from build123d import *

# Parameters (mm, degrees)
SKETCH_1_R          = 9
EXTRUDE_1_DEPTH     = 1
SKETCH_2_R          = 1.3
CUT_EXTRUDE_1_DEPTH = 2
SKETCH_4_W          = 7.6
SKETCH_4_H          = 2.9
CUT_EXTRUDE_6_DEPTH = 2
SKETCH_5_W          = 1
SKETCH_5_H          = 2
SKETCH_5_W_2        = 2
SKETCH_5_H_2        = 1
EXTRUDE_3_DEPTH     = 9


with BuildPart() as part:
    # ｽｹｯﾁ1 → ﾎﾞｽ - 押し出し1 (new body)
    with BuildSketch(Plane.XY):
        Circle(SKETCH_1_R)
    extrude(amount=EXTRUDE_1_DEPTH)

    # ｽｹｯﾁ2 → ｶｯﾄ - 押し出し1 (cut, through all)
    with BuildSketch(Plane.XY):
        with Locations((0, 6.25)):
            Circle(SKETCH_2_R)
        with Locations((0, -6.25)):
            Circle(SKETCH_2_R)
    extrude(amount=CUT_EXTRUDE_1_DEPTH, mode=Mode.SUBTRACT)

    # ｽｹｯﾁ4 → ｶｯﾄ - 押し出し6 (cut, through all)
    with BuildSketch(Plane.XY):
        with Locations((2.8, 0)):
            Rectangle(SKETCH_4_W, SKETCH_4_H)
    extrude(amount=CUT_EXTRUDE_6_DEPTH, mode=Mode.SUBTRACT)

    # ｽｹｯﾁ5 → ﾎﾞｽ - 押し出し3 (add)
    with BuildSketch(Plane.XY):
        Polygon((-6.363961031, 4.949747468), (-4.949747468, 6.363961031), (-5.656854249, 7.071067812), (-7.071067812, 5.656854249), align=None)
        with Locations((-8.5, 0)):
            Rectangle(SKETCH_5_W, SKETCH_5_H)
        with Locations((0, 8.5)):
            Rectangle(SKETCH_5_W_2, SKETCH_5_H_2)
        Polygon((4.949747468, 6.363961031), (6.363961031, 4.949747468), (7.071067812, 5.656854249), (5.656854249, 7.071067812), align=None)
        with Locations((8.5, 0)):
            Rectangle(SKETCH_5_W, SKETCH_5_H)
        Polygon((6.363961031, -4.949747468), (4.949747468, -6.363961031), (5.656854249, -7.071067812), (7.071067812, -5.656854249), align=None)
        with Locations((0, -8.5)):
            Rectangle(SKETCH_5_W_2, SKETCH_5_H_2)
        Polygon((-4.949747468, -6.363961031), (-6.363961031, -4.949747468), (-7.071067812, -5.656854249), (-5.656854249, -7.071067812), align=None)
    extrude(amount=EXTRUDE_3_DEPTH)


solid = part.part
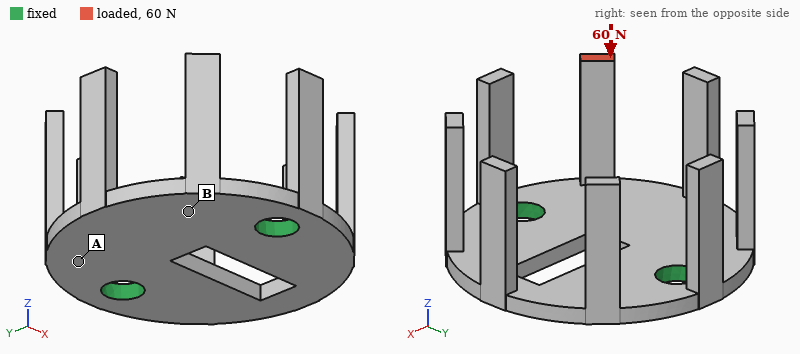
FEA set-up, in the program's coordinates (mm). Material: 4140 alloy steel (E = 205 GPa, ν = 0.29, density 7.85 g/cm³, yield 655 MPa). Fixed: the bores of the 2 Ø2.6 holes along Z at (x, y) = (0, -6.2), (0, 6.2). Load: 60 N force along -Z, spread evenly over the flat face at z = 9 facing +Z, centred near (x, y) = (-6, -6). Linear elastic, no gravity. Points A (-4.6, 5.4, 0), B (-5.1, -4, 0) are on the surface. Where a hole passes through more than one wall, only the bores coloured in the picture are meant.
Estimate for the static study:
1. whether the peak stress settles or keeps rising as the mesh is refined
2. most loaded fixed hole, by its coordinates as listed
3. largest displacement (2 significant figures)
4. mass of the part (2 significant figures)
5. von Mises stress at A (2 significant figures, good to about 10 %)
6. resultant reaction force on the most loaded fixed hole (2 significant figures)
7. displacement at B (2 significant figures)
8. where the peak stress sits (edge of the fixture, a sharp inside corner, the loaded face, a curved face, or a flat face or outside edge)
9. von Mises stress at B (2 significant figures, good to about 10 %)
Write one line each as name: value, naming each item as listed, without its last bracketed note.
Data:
whether the peak stress settles or keeps rising as the mesh is refined: keeps rising
most loaded fixed hole, by its coordinates as listed: (0, -6.2)
largest displacement: 53 µm
mass of the part: 2.7 g
von Mises stress at A: 34 MPa
resultant reaction force on the most loaded fixed hole: 59 N
displacement at B: 13 µm
where the peak stress sits: edge of the fixture
von Mises stress at B: 76 MPa
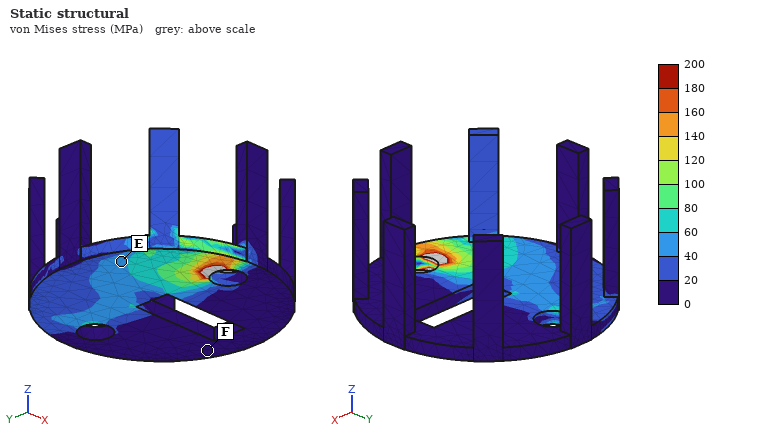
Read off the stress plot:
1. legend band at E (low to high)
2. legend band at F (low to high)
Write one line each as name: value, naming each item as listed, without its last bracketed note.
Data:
legend band at E: 40 to 60 MPa
legend band at F: 0 to 20 MPa
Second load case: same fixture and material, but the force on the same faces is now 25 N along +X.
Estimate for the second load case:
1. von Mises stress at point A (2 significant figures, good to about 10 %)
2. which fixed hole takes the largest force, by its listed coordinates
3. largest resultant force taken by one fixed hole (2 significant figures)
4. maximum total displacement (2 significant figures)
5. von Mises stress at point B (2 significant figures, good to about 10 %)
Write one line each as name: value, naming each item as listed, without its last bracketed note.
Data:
von Mises stress at point A: 39 MPa
which fixed hole takes the largest force, by its listed coordinates: (0, -6.2)
largest resultant force taken by one fixed hole: 25 N
maximum total displacement: 0.17 mm
von Mises stress at point B: 150 MPa
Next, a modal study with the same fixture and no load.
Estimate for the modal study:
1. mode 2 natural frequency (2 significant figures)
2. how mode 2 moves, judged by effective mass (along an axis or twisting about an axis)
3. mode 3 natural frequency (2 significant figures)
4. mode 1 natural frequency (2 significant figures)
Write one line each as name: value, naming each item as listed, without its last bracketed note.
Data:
mode 2 natural frequency: 6900 Hz
how mode 2 moves, judged by effective mass: along Z
mode 3 natural frequency: 8700 Hz
mode 1 natural frequency: 6600 Hz
